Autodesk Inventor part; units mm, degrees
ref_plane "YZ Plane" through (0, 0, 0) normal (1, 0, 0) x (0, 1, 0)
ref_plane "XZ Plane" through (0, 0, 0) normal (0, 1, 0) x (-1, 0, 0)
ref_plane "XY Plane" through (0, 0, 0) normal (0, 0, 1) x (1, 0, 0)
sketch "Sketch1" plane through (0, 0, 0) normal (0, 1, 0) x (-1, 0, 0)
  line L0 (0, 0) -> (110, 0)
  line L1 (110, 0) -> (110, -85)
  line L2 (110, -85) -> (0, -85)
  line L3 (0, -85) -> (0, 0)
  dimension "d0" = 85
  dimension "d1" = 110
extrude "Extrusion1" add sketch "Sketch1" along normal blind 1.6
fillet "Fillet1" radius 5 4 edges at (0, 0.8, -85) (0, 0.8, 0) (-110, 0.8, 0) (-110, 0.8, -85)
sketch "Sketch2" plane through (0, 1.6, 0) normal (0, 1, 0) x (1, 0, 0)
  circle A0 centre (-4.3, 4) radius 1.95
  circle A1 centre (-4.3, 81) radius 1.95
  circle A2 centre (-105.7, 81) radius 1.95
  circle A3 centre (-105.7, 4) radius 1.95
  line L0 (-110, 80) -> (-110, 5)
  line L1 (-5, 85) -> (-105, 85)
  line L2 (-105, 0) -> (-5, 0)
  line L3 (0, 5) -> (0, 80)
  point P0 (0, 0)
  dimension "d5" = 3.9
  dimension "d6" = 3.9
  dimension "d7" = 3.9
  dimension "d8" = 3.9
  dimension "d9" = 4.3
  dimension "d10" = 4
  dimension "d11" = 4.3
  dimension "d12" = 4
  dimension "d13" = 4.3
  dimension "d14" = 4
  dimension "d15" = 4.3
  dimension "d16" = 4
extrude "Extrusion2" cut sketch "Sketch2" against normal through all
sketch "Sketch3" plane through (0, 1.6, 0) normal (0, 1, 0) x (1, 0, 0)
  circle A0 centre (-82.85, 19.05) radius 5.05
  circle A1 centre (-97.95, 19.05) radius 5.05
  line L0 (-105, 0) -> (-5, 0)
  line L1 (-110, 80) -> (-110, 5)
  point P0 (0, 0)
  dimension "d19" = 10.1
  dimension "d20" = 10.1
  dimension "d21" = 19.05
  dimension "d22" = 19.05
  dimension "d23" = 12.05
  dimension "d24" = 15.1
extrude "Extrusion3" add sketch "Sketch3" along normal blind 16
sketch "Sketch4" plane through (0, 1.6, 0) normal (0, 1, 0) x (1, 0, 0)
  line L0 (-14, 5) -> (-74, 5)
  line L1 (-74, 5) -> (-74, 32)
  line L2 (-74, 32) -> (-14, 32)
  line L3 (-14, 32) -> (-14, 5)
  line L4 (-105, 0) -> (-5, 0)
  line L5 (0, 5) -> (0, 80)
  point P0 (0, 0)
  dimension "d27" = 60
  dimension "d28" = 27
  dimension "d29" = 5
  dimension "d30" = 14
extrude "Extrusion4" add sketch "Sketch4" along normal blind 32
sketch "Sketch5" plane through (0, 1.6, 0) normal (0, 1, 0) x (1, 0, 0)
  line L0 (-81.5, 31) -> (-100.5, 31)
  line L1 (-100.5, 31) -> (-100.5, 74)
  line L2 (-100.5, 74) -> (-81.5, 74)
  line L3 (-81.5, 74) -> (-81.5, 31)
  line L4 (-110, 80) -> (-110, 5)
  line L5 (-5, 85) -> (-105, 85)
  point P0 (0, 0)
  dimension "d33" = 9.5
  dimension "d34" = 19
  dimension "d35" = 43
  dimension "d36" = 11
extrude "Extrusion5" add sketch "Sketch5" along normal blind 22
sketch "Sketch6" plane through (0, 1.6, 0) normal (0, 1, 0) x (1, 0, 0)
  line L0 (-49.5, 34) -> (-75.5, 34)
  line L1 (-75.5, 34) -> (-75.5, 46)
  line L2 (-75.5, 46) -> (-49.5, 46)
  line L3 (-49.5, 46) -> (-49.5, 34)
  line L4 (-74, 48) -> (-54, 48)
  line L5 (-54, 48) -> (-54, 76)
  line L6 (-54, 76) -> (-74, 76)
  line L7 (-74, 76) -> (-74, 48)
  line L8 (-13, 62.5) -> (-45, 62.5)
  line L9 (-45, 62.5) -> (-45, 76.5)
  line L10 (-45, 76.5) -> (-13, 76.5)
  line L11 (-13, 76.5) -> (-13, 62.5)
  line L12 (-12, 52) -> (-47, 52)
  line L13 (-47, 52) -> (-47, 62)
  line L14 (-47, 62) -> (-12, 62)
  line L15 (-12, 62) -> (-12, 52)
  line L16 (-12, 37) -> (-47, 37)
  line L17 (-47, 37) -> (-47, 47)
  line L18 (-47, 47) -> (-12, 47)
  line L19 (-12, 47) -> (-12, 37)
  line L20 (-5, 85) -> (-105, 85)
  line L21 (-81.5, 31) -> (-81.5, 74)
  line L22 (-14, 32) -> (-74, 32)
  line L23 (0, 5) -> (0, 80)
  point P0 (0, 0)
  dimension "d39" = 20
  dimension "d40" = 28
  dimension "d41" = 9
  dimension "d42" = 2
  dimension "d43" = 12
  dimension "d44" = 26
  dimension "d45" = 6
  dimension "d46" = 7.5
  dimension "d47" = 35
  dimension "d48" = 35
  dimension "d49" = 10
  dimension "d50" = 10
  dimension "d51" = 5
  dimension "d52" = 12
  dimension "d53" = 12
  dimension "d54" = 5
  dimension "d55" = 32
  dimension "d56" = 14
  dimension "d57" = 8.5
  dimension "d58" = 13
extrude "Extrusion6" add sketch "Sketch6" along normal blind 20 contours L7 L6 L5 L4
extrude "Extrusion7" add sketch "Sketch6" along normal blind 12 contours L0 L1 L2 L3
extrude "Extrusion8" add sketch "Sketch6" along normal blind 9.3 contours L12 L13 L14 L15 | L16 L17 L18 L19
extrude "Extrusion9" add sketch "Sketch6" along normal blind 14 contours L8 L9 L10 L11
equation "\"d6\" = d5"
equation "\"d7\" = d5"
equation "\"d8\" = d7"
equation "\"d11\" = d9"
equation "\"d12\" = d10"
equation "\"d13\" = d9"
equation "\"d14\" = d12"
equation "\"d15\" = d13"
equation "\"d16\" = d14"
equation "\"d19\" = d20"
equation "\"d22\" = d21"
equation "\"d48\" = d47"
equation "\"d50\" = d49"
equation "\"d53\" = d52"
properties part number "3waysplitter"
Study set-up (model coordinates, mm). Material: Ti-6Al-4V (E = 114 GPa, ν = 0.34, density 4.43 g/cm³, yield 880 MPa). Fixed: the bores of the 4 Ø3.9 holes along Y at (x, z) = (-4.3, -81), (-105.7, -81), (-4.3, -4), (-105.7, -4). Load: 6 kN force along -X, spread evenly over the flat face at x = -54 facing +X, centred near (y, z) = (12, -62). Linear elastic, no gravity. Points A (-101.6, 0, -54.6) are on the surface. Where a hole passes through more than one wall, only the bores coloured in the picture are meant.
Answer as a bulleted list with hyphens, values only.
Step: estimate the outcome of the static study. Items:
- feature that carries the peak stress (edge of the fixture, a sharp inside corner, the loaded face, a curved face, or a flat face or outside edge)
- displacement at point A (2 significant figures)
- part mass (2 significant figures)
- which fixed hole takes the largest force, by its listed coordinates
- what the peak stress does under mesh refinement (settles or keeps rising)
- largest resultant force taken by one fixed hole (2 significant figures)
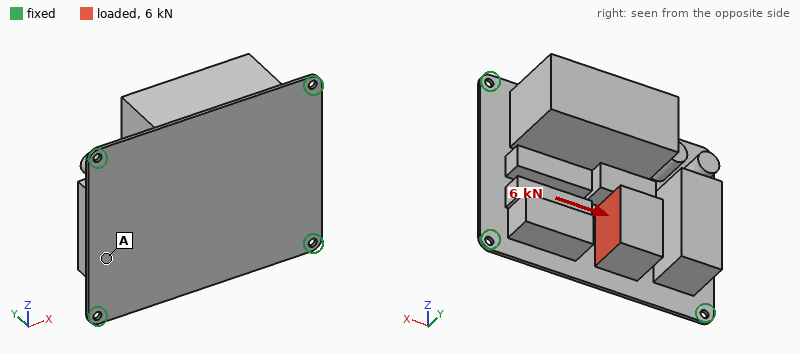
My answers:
- edge of the fixture
- 0.094 mm
- 510 g
- (-105.7, -81)
- keeps rising
- 2.1 kN
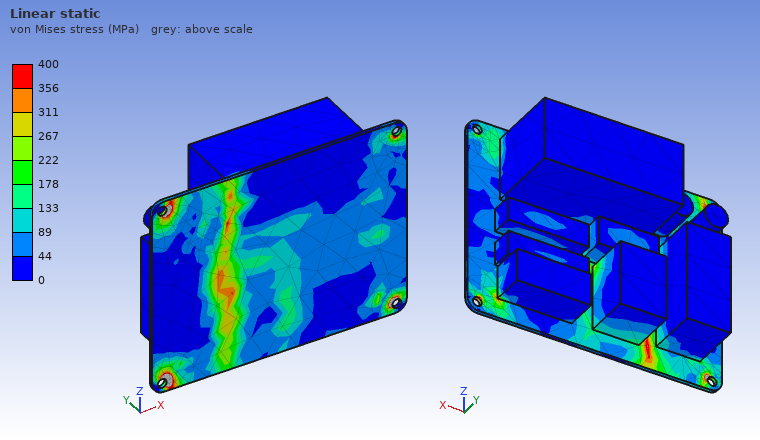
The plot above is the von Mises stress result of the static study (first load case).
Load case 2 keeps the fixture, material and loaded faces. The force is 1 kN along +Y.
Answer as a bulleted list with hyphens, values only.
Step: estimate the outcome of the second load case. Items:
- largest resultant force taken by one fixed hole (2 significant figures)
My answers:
- 460 N
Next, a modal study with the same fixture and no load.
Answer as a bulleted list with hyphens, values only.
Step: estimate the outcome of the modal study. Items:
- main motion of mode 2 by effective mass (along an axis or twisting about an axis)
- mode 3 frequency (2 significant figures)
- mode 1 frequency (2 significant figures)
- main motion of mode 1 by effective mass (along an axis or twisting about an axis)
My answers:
- along Z
- 1000 Hz
- 400 Hz
- along Y
